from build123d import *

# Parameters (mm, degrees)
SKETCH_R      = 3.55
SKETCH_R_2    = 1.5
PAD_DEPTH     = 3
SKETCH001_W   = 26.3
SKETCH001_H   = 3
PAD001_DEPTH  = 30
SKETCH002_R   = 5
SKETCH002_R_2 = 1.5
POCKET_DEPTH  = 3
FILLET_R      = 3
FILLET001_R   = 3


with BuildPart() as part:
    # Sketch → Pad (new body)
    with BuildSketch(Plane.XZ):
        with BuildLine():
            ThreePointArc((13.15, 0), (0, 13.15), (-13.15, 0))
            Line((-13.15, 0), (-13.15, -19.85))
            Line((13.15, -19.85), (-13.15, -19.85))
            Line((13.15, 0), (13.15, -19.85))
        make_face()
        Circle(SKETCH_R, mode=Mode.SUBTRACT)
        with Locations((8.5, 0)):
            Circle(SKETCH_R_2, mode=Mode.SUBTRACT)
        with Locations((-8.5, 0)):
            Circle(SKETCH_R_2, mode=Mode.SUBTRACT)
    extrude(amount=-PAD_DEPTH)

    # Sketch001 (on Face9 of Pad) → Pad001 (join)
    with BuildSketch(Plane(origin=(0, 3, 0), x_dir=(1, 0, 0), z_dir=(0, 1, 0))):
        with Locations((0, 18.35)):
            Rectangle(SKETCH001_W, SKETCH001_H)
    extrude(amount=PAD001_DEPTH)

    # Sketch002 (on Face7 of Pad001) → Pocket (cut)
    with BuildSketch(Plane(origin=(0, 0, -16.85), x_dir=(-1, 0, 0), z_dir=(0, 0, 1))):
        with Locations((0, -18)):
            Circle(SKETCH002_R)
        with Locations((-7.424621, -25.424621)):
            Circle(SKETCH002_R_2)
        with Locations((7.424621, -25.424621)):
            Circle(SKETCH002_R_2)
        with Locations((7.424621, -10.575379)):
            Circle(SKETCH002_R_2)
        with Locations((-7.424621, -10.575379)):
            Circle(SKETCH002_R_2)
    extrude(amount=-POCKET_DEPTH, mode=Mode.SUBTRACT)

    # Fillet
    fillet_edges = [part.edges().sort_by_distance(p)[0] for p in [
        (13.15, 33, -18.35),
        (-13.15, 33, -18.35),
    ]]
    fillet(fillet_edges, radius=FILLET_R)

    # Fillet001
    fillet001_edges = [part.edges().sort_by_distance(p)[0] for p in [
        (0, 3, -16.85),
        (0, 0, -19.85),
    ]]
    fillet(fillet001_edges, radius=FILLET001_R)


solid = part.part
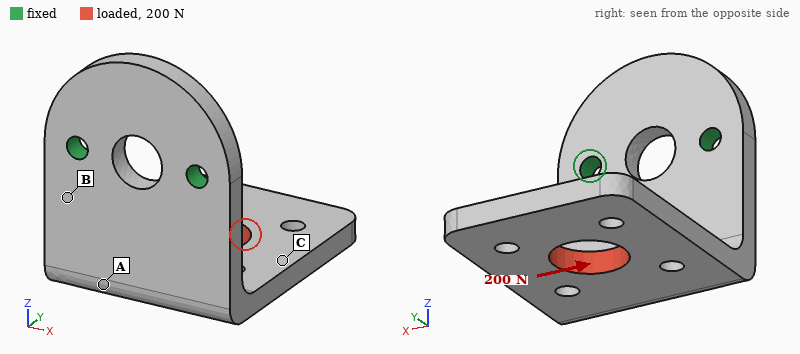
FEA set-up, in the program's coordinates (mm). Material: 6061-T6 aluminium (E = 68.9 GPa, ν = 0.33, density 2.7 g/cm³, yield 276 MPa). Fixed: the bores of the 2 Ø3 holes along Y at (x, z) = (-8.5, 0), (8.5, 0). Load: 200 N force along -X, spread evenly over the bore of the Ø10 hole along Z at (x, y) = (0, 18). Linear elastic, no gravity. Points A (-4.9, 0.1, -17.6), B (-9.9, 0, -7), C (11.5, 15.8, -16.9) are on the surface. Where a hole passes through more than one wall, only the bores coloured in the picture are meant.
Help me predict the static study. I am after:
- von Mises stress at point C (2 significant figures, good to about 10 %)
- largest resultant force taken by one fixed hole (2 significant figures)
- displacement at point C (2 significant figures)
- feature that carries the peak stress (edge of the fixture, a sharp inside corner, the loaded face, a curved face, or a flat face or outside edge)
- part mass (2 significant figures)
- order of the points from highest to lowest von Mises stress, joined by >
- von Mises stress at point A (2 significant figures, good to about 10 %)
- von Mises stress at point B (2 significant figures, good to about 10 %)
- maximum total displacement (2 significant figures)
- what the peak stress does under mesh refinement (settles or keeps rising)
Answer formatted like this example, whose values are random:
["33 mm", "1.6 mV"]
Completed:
["10 MPa", "270 N", "0.093 mm", "edge of the fixture", "11 g", "B > A > C", "28 MPa", "43 MPa", "0.17 mm", "keeps rising"]
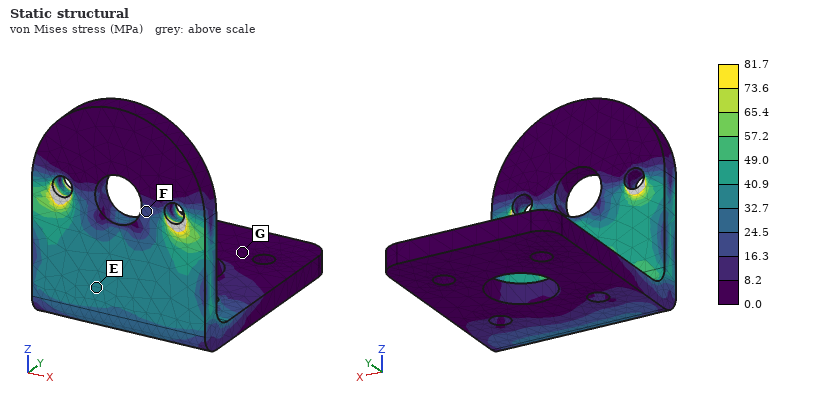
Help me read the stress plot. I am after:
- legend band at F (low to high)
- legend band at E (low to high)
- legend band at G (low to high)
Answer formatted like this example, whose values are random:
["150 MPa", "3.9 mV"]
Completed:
["16.3 to 24.5 MPa", "32.7 to 40.9 MPa", "0.0 to 8.2 MPa"]
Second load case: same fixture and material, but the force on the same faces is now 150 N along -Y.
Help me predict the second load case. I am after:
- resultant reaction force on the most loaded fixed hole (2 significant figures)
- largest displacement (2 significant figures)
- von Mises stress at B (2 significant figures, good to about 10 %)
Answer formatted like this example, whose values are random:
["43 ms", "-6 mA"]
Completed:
["75 N", "0.22 mm", "47 MPa"]
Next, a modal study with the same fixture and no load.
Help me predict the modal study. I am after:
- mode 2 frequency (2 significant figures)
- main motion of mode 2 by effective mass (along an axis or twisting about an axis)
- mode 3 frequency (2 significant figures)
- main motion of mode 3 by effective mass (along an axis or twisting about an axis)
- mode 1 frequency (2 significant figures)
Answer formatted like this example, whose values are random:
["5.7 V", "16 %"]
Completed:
["2700 Hz", "along X", "4200 Hz", "along Y", "1400 Hz"]
